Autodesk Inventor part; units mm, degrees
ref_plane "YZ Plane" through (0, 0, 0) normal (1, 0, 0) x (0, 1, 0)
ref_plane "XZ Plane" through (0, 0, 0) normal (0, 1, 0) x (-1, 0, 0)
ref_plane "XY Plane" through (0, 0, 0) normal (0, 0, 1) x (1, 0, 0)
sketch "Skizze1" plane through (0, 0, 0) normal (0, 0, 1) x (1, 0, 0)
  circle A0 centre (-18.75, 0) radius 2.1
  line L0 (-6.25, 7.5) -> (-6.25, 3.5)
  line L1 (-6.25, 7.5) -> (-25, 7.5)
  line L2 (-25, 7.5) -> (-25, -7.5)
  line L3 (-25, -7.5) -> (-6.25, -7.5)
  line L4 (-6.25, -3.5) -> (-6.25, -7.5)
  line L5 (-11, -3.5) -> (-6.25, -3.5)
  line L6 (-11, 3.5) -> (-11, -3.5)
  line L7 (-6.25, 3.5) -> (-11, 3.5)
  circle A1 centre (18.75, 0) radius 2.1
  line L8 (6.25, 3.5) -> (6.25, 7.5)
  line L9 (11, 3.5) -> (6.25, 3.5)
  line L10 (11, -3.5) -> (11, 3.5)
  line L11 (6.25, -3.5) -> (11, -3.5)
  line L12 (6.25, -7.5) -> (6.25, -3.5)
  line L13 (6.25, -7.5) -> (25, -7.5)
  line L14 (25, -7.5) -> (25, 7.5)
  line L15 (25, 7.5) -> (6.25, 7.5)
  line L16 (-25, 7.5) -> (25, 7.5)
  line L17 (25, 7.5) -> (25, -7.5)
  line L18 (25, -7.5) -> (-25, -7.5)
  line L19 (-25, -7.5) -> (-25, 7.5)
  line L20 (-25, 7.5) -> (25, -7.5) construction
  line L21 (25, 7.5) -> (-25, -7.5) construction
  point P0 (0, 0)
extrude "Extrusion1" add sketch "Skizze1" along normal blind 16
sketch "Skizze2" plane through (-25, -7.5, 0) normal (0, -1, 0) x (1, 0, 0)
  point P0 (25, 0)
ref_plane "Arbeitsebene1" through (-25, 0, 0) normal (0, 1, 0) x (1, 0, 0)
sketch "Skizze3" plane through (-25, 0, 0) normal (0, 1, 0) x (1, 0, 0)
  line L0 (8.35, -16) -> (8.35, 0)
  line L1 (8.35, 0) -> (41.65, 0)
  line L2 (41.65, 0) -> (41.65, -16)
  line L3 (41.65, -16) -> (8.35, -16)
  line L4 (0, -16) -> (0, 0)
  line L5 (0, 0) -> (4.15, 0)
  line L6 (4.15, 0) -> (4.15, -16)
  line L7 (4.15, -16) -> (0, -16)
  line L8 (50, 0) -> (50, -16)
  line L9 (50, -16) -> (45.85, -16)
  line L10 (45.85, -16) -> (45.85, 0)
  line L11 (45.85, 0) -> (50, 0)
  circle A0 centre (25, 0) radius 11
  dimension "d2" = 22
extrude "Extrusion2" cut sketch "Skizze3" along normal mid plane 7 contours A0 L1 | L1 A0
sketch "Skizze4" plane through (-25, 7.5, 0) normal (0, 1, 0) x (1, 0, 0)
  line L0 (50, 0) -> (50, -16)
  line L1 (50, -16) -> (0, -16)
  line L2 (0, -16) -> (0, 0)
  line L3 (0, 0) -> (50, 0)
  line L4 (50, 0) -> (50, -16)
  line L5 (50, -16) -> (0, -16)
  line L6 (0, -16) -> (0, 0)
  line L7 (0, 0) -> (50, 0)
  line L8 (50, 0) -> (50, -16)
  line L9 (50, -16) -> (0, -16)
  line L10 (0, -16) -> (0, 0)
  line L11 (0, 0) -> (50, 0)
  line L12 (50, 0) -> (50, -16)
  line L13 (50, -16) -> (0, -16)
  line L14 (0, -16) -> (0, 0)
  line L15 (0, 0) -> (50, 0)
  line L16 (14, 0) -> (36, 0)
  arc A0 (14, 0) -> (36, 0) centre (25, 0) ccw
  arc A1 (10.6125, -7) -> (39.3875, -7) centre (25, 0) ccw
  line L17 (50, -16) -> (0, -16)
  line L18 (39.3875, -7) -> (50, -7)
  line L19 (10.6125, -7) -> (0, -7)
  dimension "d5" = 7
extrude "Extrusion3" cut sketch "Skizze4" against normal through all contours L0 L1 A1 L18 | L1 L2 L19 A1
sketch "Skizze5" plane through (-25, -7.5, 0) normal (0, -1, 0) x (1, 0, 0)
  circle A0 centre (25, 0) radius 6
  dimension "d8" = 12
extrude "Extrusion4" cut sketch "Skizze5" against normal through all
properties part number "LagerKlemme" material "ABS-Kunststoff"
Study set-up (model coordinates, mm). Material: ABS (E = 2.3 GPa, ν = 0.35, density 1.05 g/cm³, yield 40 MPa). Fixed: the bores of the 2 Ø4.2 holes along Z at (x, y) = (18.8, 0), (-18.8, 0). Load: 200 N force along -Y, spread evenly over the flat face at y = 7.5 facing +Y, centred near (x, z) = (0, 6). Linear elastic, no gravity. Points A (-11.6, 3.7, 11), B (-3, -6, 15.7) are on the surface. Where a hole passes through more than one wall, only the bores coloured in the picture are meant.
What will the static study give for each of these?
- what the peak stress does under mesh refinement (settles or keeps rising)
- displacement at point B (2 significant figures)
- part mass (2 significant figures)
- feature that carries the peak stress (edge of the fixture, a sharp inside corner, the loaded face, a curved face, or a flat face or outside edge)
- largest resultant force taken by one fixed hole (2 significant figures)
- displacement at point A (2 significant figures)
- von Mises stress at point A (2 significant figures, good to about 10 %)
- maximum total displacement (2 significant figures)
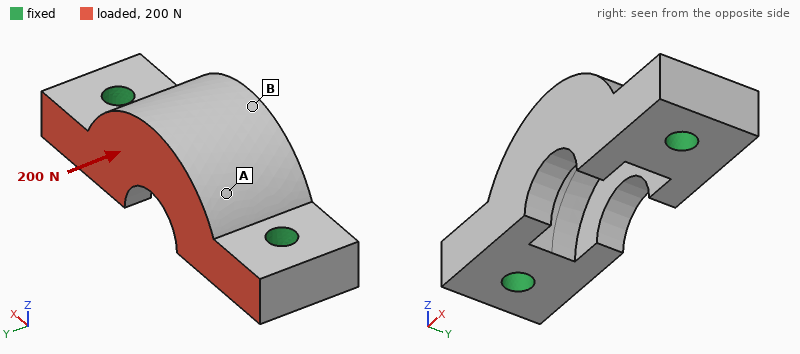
keeps rising
47 µm
6.4 g
edge of the fixture
100 N
28 µm
1.6 MPa
50 µm
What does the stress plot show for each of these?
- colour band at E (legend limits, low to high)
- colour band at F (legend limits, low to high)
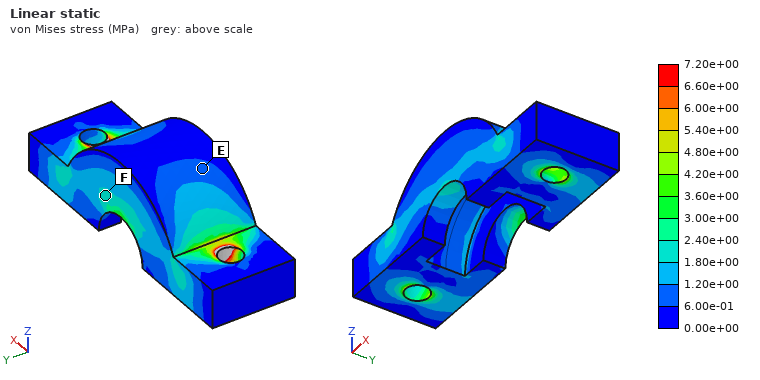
6.00e-01 to 1.20e+00 MPa
1.80e+00 to 2.40e+00 MPa
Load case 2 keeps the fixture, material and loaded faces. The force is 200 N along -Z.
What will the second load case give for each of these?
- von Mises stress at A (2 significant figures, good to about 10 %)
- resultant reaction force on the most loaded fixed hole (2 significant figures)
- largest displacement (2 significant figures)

2.1 MPa
110 N
77 µm
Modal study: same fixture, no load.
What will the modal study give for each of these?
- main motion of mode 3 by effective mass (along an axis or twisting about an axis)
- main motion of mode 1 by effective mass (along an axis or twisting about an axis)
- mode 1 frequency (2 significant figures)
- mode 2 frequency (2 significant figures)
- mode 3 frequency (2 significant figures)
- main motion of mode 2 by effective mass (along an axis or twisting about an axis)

along Y
along Y
4600 Hz
7900 Hz
10 kHz
along Z
